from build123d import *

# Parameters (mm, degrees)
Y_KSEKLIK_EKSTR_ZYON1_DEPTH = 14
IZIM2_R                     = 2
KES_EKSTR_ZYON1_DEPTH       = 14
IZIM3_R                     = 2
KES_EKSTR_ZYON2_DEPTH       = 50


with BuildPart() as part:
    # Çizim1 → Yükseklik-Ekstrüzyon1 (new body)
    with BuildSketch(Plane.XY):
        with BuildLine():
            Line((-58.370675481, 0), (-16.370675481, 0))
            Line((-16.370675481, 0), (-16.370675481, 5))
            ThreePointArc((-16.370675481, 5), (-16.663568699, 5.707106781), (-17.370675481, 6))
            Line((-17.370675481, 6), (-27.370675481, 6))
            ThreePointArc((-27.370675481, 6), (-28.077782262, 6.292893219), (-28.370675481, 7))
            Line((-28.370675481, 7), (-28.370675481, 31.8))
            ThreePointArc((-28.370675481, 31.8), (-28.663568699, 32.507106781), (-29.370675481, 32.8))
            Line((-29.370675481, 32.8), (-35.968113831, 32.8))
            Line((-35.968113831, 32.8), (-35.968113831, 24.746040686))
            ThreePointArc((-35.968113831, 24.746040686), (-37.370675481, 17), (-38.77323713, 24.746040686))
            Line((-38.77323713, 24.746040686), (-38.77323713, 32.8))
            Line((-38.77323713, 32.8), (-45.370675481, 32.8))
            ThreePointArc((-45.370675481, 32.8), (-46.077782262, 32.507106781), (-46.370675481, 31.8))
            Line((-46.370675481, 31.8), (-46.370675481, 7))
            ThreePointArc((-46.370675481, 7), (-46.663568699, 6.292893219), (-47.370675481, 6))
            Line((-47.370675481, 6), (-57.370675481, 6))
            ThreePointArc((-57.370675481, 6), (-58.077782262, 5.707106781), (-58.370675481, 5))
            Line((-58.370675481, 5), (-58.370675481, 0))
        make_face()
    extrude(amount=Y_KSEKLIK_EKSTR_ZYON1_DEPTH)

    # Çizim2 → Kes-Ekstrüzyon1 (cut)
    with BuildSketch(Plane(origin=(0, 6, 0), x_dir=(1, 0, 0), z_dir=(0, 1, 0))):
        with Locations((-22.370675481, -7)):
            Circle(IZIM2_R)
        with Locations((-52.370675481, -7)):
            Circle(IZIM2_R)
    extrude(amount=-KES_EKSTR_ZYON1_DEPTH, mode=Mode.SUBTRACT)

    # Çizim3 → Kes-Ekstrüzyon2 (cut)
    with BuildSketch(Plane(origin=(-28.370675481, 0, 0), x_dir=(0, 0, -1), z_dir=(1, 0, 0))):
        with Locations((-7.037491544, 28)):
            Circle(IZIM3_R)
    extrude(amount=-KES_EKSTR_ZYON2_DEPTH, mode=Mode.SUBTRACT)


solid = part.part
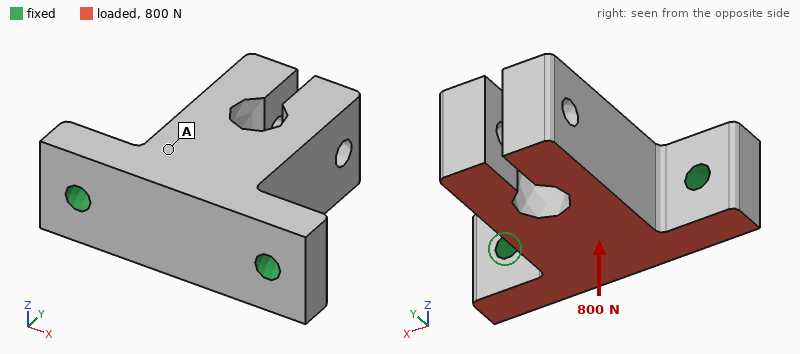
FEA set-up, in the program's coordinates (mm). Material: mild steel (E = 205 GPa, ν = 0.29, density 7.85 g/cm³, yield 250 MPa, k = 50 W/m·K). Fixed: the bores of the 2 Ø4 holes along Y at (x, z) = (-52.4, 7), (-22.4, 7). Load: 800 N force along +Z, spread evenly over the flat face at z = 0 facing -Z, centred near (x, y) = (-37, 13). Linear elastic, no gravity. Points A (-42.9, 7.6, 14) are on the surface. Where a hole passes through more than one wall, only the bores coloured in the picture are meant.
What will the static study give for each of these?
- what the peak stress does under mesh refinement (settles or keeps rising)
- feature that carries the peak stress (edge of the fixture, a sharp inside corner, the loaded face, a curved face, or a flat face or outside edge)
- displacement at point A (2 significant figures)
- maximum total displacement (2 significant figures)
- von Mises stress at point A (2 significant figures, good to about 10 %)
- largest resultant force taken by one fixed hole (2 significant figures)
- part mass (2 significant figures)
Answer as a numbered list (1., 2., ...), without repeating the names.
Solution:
1. keeps rising
2. edge of the fixture
3. 4.1 µm
4. 16 µm
5. 8.3 MPa
6. 400 N
7. 70 g
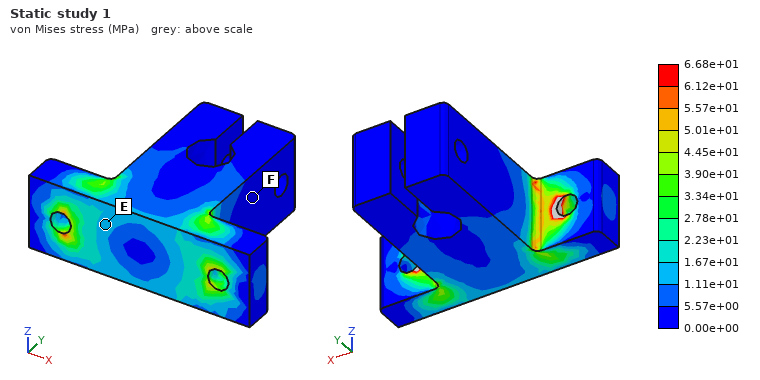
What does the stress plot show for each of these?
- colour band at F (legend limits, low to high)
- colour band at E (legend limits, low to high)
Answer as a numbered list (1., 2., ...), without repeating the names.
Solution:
1. 0.00e+00 to 5.57e+00 MPa
2. 1.11e+01 to 1.67e+01 MPa
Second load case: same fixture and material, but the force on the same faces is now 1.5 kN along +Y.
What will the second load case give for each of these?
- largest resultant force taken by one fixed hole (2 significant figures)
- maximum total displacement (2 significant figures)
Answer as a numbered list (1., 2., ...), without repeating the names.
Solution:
1. 780 N
2. 18 µm
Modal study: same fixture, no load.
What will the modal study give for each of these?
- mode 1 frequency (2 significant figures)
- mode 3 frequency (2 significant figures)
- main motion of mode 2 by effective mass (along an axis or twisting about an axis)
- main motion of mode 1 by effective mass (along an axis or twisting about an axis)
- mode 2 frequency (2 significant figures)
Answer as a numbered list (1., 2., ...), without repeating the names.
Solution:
1. 5300 Hz
2. 12 kHz
3. along X
4. along Z
5. 9300 Hz
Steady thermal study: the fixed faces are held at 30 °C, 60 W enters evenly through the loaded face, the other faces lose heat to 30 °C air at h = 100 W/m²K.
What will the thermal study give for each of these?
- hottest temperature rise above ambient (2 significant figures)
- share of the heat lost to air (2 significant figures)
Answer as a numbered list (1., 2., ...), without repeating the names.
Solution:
1. 75 K
2. 23 %
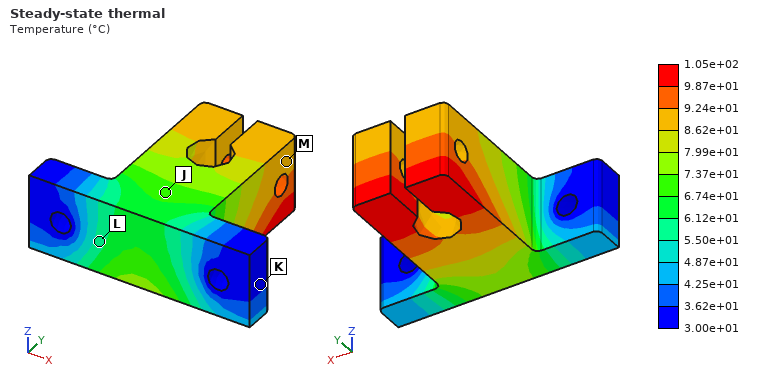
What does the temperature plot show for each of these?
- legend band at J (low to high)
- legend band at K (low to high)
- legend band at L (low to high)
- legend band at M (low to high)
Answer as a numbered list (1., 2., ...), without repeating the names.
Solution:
1. 6.74e+01 to 7.37e+01 °C
2. 3.00e+01 to 3.62e+01 °C
3. 5.50e+01 to 6.12e+01 °C
4. 8.62e+01 to 9.24e+01 °C
